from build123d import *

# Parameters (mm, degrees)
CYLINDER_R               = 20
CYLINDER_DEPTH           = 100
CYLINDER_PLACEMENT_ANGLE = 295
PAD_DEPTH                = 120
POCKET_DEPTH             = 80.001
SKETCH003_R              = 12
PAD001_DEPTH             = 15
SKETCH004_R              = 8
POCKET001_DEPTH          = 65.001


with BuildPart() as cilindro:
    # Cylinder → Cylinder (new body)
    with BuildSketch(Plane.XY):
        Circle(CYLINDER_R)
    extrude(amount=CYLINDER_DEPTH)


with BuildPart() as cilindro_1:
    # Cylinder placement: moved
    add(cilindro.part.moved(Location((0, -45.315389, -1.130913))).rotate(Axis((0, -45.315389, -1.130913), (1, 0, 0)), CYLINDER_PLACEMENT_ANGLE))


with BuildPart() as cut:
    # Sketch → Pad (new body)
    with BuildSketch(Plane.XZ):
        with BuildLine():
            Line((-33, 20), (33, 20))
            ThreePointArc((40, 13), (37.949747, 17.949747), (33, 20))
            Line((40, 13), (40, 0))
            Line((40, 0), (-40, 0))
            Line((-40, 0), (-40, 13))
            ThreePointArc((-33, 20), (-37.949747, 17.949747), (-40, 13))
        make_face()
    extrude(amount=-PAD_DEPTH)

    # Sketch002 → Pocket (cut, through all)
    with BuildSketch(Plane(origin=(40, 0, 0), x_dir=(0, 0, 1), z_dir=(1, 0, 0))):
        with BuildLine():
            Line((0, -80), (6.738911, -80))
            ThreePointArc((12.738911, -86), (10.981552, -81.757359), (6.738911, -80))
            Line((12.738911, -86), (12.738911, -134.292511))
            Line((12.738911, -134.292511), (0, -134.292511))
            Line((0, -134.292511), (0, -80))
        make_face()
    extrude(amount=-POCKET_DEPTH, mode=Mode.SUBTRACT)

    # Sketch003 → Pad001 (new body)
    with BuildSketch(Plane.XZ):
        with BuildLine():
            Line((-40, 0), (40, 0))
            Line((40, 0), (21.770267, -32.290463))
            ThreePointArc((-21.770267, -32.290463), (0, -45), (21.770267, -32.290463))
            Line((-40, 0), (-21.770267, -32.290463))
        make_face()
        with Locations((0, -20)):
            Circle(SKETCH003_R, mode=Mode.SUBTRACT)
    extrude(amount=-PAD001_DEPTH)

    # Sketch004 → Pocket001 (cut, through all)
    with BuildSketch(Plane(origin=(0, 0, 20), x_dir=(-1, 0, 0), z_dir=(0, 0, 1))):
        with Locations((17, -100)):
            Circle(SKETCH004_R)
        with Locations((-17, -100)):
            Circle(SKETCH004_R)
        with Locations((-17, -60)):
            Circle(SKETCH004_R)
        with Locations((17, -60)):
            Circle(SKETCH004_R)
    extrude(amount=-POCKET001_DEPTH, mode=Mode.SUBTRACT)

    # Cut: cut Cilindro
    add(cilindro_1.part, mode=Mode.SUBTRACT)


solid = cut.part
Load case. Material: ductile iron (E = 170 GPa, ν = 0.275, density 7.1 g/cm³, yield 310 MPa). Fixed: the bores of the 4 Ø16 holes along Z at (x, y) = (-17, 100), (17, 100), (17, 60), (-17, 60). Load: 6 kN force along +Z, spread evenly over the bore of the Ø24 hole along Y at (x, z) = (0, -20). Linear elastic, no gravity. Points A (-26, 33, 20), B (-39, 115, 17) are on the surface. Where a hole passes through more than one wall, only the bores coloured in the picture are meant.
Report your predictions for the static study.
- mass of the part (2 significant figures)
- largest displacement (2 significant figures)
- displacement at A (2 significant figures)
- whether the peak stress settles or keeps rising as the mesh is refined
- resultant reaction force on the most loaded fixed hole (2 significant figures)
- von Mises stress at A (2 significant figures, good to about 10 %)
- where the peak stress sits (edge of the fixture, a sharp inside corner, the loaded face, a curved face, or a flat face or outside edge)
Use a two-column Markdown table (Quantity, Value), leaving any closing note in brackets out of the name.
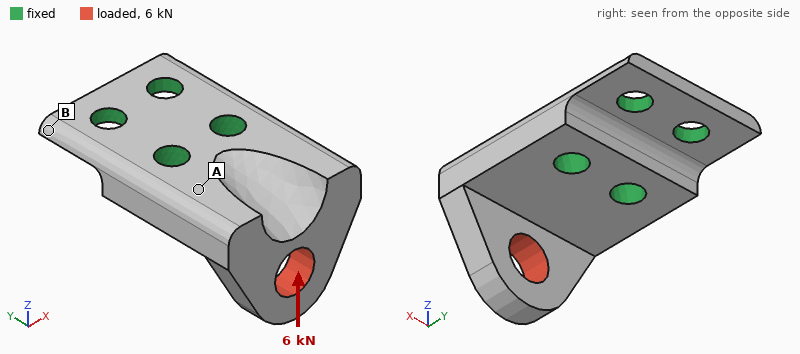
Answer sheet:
| Quantity | Value |
|---|---|
| mass of the part | 1.1 kg |
| largest displacement | 68 µm |
| displacement at A | 11 µm |
| whether the peak stress settles or keeps rising as the mesh is refined | keeps rising |
| resultant reaction force on the most loaded fixed hole | 3.2 kN |
| von Mises stress at A | 36 MPa |
| where the peak stress sits | edge of the fixture |
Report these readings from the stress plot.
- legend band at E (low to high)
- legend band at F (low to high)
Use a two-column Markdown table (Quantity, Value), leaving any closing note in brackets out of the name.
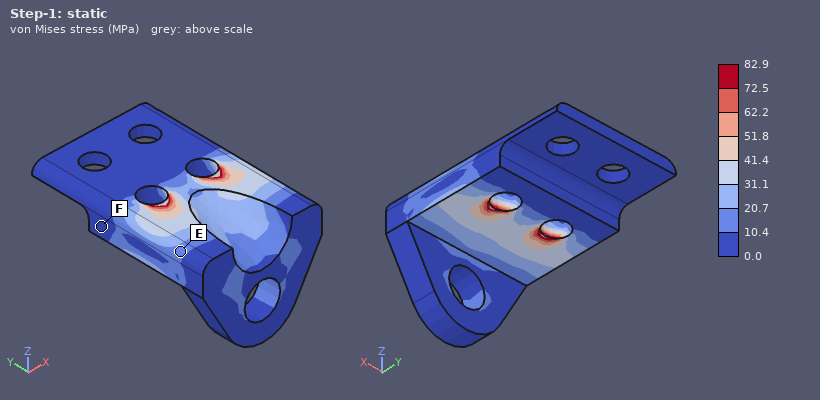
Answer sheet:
| Quantity | Value |
|---|---|
| legend band at E | 10.4 to 20.7 MPa |
| legend band at F | 0.0 to 10.4 MPa |
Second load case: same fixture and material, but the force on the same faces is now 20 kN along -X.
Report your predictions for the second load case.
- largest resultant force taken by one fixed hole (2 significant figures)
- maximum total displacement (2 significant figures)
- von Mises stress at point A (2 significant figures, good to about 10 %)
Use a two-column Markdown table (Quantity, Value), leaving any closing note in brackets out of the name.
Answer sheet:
| Quantity | Value |
|---|---|
| largest resultant force taken by one fixed hole | 23 kN |
| maximum total displacement | 0.13 mm |
| von Mises stress at point A | 69 MPa |
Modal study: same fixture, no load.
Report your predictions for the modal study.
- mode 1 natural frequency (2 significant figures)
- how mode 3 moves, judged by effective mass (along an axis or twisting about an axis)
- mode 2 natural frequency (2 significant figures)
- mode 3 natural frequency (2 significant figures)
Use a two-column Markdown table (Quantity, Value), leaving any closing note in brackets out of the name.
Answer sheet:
| Quantity | Value |
|---|---|
| mode 1 natural frequency | 2700 Hz |
| how mode 3 moves, judged by effective mass | along Z |
| mode 2 natural frequency | 4200 Hz |
| mode 3 natural frequency | 5800 Hz |
